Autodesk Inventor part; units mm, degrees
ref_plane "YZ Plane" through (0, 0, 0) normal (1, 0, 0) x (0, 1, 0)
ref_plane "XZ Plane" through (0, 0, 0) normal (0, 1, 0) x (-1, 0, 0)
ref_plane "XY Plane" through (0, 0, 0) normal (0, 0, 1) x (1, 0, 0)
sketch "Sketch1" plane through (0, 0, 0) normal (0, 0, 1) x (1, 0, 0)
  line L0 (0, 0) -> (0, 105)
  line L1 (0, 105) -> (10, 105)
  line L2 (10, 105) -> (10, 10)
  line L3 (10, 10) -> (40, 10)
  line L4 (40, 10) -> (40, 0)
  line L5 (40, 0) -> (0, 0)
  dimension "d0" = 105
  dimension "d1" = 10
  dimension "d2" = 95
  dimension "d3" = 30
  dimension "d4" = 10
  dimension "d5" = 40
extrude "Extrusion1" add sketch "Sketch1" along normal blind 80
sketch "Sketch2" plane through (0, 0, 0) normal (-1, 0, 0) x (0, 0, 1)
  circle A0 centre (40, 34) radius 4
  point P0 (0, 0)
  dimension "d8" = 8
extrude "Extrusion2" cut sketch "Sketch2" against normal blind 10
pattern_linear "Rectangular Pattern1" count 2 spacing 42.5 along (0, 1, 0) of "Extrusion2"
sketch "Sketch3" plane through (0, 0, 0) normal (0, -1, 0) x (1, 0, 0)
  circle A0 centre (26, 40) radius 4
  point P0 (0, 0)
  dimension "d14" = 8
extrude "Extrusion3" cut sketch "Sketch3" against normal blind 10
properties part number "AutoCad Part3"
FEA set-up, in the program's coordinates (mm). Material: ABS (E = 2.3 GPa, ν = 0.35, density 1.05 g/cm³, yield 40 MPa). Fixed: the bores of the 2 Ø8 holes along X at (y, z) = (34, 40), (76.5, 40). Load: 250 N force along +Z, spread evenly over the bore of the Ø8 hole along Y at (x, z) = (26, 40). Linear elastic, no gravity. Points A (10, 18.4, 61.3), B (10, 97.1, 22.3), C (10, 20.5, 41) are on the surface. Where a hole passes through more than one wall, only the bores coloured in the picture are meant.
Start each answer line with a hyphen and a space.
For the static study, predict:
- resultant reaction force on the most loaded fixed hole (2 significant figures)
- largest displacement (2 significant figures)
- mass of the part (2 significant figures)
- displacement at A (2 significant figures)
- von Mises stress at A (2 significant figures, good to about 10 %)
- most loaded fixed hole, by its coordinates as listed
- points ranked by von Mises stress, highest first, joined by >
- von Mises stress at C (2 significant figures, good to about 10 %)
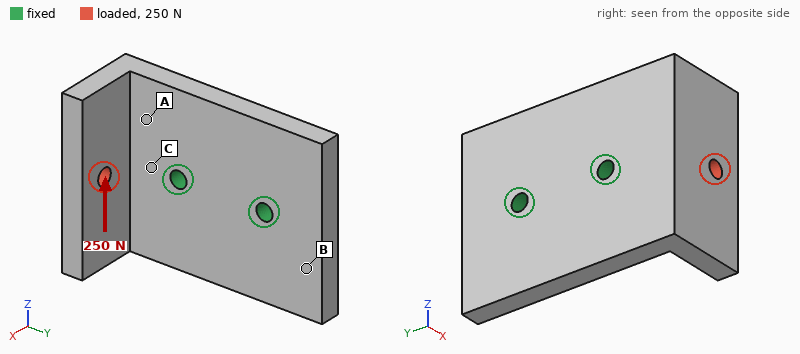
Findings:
- 390 N
- 0.39 mm
- 110 g
- 0.12 mm
- 2.1 MPa
- (34, 40)
- C > A > B
- 3.4 MPa
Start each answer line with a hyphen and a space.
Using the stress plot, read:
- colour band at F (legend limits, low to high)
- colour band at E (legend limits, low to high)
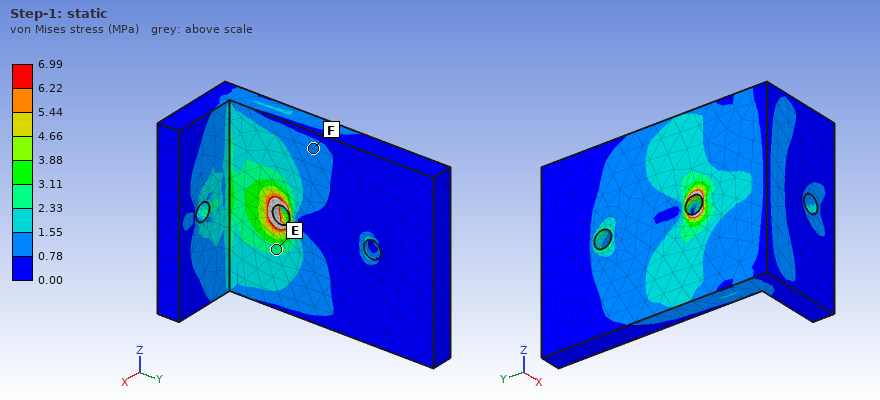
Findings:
- 0.78 to 1.55 MPa
- 2.33 to 3.11 MPa
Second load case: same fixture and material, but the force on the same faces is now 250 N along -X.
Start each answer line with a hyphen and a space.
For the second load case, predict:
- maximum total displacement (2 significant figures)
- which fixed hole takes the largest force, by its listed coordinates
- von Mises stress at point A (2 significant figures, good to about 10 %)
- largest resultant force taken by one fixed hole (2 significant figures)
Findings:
- 0.40 mm
- (34, 40)
- 2.2 MPa
- 320 N
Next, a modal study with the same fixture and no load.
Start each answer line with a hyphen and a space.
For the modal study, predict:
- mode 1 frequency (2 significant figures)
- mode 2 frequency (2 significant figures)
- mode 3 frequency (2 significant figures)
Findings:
- 700 Hz
- 710 Hz
- 1300 Hz
